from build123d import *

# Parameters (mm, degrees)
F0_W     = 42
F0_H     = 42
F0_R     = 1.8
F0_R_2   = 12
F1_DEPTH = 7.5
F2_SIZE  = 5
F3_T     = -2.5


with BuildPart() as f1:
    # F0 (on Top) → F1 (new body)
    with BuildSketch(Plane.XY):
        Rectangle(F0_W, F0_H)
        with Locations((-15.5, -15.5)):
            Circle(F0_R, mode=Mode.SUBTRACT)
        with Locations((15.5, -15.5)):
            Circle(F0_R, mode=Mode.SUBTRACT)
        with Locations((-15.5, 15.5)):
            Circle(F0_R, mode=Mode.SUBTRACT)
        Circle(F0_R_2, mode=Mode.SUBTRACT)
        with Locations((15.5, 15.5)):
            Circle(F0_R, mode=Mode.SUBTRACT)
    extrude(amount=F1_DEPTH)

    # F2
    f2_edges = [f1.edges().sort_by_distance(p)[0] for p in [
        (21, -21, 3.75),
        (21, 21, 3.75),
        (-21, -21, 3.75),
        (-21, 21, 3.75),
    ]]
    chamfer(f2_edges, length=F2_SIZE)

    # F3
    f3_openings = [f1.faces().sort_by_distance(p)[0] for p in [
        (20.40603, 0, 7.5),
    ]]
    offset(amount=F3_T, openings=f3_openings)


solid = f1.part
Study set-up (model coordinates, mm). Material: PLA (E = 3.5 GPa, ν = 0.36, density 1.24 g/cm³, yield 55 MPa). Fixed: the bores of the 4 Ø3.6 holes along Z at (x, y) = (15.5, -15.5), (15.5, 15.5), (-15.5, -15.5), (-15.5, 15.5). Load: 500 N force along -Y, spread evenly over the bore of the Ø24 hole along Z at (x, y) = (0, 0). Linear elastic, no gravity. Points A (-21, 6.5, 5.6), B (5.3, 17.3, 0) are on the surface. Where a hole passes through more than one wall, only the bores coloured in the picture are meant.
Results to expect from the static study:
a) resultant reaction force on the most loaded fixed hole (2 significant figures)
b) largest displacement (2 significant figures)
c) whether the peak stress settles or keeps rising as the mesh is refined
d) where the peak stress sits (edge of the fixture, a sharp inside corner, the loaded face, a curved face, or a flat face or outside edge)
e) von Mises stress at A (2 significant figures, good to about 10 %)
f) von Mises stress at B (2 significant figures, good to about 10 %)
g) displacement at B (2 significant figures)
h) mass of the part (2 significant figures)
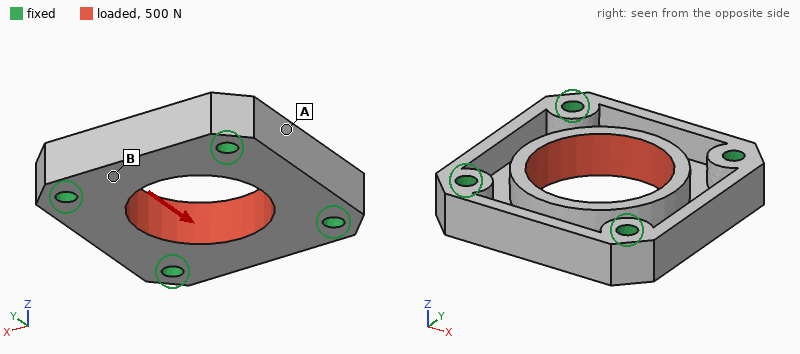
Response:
130 N
50 µm
keeps rising
edge of the fixture
1.1 MPa
2.5 MPa
22 µm
8.1 g
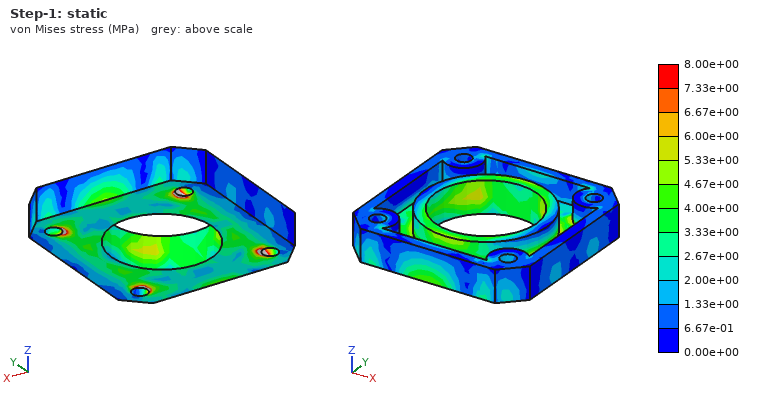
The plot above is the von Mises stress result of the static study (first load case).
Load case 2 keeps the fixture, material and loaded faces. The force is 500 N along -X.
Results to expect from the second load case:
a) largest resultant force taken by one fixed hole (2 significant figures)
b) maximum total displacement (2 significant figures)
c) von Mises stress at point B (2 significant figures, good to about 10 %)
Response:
130 N
50 µm
2.2 MPa
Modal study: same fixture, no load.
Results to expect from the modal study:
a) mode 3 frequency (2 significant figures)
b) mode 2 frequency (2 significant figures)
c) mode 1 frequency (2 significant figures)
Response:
8600 Hz
7700 Hz
7600 Hz
